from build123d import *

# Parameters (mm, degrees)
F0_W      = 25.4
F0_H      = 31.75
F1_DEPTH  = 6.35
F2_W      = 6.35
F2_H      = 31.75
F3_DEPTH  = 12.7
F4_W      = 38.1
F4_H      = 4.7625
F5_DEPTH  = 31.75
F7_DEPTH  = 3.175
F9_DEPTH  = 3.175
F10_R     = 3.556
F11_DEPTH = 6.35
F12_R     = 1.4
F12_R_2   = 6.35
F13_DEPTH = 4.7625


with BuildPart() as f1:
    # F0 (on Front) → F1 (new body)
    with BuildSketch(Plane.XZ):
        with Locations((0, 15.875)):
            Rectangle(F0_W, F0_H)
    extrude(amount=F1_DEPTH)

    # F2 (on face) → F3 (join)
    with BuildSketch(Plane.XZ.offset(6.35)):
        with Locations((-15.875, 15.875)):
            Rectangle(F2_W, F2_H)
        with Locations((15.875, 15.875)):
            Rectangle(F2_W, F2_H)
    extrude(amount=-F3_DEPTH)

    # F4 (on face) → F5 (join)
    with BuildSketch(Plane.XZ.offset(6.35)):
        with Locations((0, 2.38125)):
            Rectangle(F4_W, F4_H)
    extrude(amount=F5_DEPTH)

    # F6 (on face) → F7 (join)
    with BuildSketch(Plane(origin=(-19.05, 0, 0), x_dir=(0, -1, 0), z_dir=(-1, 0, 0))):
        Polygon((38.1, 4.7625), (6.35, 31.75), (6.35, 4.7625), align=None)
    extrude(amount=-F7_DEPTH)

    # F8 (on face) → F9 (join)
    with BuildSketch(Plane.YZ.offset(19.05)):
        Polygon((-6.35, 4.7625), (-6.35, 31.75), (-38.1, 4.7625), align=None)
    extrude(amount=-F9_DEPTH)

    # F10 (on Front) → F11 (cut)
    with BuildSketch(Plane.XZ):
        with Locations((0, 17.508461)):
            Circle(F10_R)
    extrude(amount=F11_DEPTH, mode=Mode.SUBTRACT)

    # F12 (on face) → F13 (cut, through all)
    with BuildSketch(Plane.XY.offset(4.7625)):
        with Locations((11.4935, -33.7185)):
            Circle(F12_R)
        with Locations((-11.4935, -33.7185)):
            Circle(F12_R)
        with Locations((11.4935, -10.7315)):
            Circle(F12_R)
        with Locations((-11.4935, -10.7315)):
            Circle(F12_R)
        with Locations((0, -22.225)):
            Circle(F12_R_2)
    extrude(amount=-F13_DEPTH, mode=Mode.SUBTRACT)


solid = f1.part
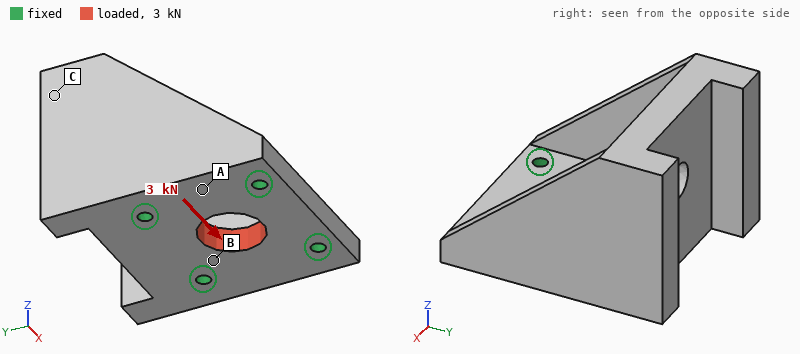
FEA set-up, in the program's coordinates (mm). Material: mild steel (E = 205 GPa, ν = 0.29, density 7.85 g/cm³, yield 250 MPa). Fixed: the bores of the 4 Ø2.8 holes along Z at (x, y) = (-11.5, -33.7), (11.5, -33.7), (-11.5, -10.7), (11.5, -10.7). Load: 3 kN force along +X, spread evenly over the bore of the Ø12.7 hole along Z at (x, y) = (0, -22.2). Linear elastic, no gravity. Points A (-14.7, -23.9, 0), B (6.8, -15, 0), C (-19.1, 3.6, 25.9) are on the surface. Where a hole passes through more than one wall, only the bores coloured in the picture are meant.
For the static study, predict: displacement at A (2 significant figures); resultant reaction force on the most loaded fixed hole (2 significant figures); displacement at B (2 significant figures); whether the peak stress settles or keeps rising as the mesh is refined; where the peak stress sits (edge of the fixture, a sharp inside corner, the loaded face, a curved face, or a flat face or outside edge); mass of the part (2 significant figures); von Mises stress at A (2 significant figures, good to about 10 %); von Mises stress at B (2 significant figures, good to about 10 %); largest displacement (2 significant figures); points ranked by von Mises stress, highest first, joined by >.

0.94 µm
780 N
0.64 µm
keeps rising
edge of the fixture
140 g
6.8 MPa
16 MPa
1.4 µm
B > A > C
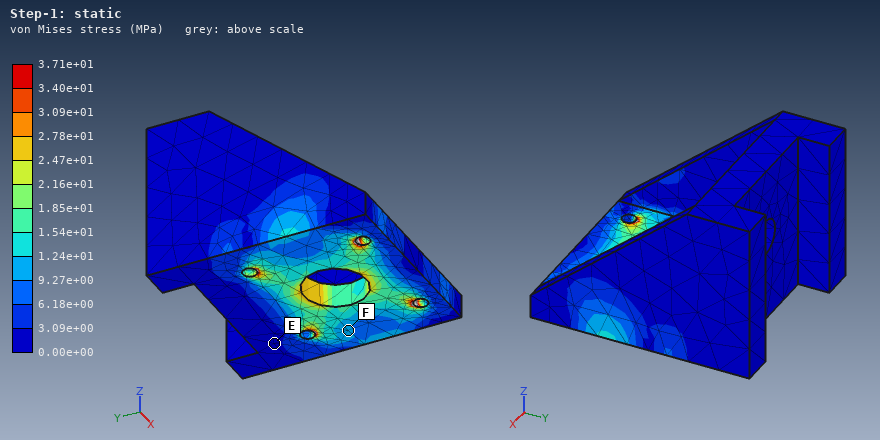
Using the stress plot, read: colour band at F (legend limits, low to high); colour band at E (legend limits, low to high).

9.27e+00 to 1.24e+01 MPa
0.00e+00 to 3.09e+00 MPa
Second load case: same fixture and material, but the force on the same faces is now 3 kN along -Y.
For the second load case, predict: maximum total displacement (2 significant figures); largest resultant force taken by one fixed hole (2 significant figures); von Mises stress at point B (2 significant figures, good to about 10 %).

1.6 µm
800 N
16 MPa
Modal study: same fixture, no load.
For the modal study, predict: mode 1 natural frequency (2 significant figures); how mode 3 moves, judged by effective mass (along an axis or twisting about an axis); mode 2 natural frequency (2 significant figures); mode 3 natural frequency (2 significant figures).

7100 Hz
along X
7300 Hz
14 kHz
